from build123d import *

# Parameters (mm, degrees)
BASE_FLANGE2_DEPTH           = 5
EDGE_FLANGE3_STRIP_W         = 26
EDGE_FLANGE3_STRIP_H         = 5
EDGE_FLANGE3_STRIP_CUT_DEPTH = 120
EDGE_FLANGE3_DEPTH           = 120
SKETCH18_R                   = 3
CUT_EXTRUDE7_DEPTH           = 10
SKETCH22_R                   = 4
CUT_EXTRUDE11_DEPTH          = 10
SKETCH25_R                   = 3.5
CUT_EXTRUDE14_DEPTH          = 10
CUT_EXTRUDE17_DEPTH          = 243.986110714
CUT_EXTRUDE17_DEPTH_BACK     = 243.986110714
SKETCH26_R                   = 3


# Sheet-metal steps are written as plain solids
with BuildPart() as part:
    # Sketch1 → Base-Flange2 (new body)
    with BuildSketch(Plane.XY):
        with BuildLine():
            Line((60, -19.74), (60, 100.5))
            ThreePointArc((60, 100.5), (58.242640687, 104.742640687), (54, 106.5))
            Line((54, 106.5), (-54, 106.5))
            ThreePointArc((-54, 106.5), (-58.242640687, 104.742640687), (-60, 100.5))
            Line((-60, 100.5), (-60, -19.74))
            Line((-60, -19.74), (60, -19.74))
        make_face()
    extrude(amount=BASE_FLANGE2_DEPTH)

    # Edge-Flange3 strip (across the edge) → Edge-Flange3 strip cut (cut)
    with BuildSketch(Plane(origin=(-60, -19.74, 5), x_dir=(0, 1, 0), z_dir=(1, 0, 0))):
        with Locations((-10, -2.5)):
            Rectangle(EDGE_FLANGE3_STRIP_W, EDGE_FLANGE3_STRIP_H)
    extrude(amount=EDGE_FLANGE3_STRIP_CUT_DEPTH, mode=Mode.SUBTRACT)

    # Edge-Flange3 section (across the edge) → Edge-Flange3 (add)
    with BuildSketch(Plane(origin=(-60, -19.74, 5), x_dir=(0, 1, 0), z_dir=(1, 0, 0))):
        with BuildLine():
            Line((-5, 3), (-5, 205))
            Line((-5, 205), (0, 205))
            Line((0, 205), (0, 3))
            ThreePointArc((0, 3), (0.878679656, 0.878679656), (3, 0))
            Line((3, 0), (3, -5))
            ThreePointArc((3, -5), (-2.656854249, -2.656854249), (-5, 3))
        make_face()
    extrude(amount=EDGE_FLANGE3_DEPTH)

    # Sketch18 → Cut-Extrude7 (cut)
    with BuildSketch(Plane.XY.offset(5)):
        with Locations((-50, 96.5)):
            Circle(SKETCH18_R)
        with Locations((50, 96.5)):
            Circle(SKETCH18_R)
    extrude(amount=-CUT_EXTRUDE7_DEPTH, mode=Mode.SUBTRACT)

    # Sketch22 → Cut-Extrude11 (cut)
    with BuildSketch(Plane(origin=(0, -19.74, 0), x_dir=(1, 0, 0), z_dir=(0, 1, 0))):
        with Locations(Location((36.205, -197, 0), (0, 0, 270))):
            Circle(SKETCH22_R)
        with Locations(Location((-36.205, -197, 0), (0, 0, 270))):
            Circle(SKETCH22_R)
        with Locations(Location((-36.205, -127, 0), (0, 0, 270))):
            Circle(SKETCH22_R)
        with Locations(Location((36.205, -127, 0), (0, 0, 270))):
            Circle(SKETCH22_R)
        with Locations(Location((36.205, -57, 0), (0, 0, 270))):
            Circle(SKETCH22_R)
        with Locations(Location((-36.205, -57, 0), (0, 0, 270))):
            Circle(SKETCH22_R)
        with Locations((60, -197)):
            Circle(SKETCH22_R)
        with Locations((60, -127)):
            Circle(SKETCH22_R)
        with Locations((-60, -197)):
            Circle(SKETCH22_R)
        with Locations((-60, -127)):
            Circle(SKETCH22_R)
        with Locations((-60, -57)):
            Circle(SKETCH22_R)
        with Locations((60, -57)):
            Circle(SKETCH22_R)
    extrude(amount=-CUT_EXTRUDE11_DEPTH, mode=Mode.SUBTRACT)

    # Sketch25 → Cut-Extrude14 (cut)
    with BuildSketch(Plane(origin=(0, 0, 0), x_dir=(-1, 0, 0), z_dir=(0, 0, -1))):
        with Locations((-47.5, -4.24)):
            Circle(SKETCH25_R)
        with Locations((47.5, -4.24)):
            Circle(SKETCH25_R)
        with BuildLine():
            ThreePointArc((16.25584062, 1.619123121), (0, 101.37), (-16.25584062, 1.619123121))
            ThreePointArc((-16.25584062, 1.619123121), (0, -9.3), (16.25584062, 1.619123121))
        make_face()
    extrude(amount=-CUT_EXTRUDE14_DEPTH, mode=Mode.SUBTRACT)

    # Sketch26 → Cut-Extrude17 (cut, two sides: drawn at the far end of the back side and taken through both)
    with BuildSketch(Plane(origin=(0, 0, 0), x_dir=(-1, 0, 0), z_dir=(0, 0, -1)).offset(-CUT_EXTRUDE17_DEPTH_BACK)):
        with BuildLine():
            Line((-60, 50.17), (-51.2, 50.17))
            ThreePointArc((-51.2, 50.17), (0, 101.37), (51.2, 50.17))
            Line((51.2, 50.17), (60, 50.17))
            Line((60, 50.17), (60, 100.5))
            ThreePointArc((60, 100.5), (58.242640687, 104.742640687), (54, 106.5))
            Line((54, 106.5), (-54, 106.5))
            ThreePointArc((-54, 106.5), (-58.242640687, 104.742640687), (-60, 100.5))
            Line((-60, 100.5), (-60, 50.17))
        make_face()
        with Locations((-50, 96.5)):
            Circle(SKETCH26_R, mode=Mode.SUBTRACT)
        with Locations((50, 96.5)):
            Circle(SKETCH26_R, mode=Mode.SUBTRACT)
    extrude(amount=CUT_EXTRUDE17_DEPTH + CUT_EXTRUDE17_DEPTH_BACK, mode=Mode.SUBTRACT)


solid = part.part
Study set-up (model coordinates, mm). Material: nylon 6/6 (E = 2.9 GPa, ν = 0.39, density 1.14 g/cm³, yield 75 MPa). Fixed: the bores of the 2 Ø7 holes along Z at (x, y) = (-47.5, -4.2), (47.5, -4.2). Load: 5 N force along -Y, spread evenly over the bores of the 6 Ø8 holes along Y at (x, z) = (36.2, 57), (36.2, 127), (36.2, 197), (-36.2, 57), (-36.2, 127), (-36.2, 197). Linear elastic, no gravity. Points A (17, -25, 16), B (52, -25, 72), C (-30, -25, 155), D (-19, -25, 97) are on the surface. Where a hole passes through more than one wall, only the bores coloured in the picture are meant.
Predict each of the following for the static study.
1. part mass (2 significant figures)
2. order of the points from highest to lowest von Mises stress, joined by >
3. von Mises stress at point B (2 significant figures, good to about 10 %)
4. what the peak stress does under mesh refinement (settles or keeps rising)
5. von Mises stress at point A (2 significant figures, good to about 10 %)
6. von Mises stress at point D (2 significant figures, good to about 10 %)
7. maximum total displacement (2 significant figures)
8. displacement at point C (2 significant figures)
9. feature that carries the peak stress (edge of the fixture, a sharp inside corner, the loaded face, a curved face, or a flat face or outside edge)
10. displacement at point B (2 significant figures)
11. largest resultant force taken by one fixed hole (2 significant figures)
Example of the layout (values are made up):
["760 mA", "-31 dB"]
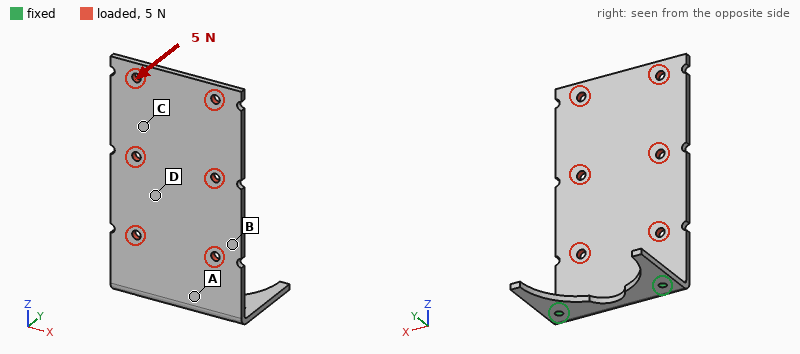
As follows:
["160 g", "A > B > D > C", "0.61 MPa", "keeps rising", "0.94 MPa", "0.41 MPa", "2.7 mm", "1.8 mm", "edge of the fixture", "0.56 mm", "4.0 N"]
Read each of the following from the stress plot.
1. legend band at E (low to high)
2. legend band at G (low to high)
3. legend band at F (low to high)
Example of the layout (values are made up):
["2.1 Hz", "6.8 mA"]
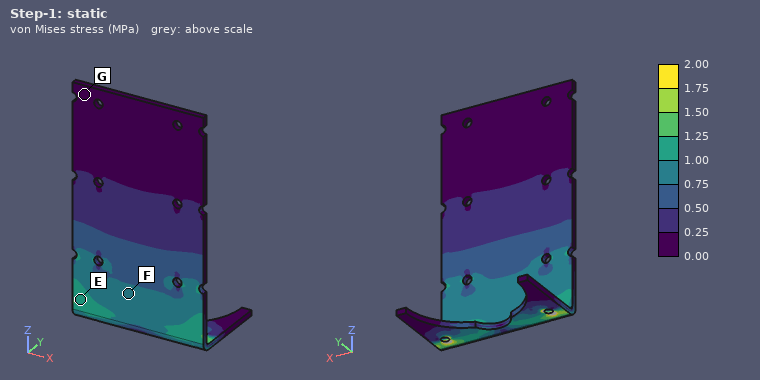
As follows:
["1.00 to 1.25 MPa", "0.00 to 0.25 MPa", "0.75 to 1.00 MPa"]
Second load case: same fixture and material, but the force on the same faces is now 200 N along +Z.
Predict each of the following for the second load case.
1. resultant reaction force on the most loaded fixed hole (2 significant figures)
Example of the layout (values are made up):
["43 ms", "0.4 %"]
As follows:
["100 N"]
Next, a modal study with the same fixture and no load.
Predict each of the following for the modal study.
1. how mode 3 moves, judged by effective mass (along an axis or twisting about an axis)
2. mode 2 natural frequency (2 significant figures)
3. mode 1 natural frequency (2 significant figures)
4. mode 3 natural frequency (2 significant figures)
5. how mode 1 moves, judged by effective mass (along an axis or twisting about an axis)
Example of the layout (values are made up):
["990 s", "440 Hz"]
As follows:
["along Y", "110 Hz", "26 Hz", "160 Hz", "along Y"]
